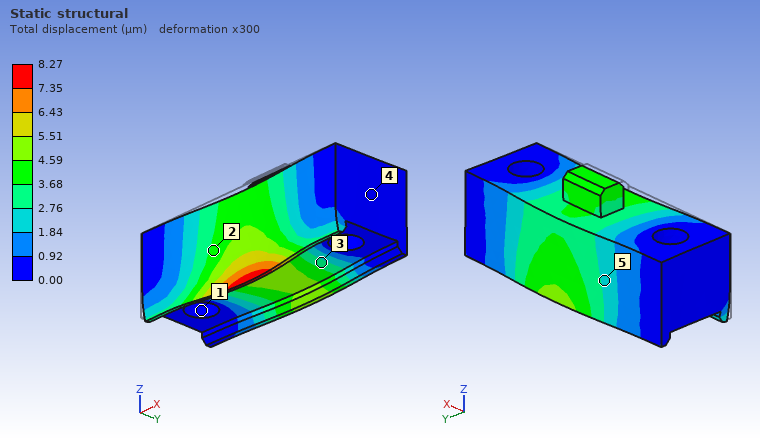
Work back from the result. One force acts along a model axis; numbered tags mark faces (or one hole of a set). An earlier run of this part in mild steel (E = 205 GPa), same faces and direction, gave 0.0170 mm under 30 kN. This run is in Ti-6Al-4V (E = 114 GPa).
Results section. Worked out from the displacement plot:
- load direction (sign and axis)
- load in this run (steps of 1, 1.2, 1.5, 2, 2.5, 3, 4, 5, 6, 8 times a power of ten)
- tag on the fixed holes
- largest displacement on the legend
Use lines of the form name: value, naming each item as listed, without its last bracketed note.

load direction: +Y
load in this run: 8 kN
tag on the fixed holes: 1
largest displacement on the legend: 8.27 µm
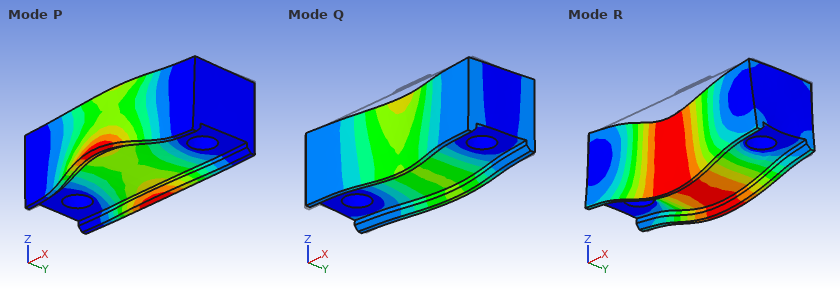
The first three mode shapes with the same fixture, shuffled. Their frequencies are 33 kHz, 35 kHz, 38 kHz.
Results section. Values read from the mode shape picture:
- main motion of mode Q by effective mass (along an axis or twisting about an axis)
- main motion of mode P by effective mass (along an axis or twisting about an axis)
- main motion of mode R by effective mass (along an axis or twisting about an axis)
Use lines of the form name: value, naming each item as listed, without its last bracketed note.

main motion of mode Q by effective mass: along Y
main motion of mode P by effective mass: twisting about X
main motion of mode R by effective mass: along Z
